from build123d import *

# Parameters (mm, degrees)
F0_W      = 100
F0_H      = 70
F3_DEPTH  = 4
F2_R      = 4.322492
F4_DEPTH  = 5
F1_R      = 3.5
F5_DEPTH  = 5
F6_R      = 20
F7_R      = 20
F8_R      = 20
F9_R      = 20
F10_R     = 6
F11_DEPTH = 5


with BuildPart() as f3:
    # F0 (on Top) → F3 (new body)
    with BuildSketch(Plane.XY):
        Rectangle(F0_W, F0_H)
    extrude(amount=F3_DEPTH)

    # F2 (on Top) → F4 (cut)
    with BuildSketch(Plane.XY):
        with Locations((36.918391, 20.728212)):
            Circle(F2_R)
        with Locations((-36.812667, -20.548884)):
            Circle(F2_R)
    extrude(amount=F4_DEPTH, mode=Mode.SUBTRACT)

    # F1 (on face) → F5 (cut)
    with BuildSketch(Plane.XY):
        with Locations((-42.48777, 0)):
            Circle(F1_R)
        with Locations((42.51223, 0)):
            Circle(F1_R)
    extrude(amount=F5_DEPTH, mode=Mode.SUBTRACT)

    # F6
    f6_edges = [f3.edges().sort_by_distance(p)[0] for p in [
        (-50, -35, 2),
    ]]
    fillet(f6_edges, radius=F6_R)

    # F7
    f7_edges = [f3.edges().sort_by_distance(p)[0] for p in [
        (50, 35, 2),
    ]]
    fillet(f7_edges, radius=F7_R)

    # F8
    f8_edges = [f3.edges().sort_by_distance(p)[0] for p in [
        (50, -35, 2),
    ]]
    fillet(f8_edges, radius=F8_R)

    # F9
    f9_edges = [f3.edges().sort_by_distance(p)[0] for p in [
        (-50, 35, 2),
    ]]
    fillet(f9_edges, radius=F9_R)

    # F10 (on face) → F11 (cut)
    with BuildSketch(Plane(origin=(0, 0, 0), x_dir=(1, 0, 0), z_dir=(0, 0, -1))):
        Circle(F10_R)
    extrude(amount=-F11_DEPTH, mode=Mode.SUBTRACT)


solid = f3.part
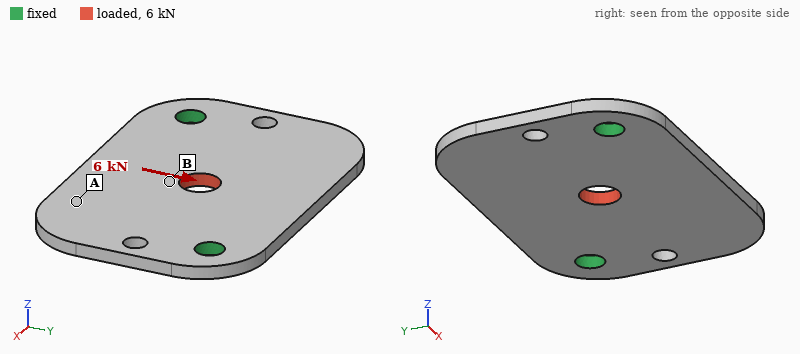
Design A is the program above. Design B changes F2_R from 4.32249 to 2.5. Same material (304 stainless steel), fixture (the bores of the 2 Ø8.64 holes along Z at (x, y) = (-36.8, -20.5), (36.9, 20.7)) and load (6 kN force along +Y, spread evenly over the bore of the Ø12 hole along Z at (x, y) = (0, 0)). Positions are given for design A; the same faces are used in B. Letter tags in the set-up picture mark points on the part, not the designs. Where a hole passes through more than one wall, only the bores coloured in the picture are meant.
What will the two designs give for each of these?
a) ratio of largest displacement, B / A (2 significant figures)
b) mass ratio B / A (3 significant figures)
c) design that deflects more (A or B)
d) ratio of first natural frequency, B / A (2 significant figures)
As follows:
1.1
1.01
B
0.89
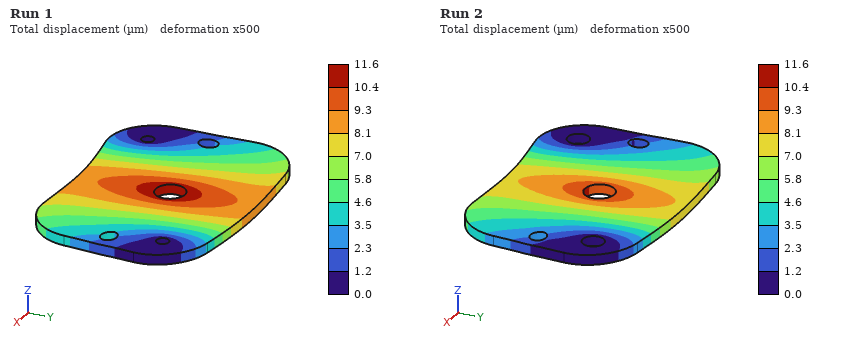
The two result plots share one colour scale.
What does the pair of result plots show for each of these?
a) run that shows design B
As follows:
Run 1
